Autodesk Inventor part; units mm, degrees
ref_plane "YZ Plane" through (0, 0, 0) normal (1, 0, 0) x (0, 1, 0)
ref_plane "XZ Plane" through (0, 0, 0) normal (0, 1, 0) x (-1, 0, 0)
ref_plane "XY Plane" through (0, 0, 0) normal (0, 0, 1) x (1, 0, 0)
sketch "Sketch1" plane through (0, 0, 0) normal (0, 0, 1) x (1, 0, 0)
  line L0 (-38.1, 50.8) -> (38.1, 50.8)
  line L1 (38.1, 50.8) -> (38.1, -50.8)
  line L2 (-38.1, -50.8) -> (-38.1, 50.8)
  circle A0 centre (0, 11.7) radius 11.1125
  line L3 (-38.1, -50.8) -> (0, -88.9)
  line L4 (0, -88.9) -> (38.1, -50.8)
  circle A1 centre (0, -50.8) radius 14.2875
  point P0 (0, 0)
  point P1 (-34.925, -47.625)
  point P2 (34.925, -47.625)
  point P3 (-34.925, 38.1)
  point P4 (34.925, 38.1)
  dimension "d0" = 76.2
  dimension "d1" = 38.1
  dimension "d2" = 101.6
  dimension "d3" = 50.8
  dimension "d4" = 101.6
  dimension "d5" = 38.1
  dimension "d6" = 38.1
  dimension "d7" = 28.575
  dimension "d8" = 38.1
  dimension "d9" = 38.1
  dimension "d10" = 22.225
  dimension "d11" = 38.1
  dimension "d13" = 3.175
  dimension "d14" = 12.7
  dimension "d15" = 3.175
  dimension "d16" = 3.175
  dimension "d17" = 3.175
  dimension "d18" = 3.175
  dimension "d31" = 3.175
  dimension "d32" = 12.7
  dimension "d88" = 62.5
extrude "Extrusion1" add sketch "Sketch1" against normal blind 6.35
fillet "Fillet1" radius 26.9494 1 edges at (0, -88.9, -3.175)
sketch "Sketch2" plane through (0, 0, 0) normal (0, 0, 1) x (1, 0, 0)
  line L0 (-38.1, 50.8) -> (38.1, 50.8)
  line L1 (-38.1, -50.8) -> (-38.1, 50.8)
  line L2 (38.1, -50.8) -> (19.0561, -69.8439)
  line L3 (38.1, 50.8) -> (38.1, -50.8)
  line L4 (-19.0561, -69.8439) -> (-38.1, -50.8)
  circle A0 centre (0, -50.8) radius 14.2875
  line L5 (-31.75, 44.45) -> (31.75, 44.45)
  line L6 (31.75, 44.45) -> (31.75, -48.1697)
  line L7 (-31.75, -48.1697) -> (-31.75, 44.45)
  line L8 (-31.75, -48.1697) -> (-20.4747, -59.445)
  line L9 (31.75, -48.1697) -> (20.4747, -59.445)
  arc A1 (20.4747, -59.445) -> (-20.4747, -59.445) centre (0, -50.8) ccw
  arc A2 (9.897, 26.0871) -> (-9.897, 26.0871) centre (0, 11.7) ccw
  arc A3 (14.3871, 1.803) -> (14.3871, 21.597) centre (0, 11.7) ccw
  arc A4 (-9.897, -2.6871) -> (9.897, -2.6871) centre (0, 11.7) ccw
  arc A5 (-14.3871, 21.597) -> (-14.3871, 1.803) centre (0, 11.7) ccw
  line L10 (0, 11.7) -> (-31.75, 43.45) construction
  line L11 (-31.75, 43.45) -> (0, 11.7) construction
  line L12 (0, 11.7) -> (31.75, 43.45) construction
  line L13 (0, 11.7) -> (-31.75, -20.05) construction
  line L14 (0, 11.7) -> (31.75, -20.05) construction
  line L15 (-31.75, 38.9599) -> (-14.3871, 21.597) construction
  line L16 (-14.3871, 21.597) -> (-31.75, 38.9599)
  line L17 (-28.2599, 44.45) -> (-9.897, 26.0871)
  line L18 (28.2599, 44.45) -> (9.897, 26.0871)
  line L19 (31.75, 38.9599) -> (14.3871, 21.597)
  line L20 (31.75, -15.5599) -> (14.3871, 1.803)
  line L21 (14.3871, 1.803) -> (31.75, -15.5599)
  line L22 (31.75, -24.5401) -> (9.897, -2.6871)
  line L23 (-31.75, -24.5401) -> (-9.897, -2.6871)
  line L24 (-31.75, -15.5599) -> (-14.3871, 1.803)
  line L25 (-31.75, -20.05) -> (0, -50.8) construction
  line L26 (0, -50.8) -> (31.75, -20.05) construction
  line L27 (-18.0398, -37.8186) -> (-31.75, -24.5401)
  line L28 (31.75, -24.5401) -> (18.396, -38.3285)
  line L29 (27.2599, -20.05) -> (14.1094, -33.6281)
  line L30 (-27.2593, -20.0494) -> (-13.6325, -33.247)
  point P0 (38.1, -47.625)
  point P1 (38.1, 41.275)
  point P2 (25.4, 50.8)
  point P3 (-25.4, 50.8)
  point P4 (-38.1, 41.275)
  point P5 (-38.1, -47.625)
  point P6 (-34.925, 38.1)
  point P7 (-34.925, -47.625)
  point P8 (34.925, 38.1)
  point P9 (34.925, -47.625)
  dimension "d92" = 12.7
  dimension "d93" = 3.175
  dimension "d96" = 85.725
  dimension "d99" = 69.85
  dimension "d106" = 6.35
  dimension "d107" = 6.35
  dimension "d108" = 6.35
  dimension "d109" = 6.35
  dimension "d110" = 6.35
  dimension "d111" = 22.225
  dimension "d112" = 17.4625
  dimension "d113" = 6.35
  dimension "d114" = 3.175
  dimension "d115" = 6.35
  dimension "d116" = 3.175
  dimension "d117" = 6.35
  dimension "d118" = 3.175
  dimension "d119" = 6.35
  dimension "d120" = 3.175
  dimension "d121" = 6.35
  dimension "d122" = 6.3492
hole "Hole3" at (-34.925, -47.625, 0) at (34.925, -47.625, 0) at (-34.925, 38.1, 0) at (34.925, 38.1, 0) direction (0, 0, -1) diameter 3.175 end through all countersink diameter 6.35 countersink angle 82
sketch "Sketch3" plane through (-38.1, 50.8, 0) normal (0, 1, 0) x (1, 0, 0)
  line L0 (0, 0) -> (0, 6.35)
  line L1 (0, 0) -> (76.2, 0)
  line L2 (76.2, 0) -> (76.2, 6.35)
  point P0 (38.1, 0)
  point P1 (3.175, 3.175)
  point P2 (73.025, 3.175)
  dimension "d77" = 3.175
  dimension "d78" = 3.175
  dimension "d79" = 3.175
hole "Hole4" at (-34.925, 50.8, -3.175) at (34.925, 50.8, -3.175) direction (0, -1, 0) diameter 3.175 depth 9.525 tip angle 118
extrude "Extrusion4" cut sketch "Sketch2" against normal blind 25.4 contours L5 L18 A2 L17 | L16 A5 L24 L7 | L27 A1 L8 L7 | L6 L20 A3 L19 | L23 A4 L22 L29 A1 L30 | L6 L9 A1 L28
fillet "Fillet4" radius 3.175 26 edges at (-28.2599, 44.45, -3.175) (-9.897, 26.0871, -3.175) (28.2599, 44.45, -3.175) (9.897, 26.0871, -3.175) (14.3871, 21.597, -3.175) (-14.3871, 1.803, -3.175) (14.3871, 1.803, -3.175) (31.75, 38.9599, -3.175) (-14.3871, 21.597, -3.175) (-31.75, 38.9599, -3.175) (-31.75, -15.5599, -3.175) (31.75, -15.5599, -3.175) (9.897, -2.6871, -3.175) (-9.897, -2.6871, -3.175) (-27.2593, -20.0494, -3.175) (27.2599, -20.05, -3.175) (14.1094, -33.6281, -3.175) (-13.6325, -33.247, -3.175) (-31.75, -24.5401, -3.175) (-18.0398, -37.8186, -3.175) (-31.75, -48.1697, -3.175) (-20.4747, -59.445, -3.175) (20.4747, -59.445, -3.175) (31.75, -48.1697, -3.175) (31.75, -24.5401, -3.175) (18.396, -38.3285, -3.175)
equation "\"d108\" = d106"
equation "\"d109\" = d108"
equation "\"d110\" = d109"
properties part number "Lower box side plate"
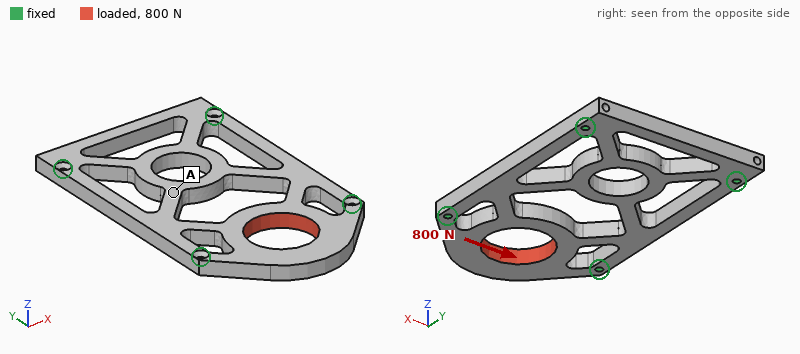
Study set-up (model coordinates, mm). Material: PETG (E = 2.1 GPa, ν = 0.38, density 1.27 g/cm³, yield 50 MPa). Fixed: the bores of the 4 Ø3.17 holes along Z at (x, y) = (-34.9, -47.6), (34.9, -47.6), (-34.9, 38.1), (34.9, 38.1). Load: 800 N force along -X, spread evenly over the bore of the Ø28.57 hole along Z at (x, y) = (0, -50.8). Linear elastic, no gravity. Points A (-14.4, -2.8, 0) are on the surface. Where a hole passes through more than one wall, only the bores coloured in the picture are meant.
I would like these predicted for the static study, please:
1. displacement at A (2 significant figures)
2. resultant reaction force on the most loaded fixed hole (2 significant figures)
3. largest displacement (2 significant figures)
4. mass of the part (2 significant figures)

0.17 mm
370 N
0.31 mm
38 g
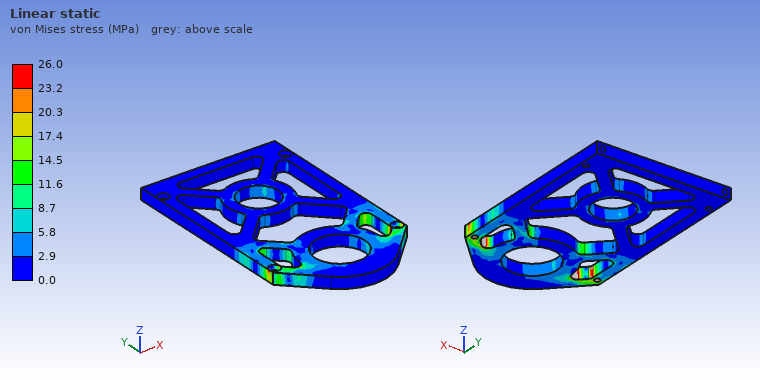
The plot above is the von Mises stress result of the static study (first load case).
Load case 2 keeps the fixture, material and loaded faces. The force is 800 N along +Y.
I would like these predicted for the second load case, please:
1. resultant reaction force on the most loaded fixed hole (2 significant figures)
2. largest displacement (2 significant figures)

410 N
0.26 mm
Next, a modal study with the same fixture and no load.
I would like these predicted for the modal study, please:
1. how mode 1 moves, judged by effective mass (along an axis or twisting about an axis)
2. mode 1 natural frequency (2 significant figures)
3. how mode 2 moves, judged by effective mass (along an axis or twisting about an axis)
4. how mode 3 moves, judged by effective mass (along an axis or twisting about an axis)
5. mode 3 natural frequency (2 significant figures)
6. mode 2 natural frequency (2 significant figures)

along Z
670 Hz
along Z
twisting about Y
1100 Hz
750 Hz
